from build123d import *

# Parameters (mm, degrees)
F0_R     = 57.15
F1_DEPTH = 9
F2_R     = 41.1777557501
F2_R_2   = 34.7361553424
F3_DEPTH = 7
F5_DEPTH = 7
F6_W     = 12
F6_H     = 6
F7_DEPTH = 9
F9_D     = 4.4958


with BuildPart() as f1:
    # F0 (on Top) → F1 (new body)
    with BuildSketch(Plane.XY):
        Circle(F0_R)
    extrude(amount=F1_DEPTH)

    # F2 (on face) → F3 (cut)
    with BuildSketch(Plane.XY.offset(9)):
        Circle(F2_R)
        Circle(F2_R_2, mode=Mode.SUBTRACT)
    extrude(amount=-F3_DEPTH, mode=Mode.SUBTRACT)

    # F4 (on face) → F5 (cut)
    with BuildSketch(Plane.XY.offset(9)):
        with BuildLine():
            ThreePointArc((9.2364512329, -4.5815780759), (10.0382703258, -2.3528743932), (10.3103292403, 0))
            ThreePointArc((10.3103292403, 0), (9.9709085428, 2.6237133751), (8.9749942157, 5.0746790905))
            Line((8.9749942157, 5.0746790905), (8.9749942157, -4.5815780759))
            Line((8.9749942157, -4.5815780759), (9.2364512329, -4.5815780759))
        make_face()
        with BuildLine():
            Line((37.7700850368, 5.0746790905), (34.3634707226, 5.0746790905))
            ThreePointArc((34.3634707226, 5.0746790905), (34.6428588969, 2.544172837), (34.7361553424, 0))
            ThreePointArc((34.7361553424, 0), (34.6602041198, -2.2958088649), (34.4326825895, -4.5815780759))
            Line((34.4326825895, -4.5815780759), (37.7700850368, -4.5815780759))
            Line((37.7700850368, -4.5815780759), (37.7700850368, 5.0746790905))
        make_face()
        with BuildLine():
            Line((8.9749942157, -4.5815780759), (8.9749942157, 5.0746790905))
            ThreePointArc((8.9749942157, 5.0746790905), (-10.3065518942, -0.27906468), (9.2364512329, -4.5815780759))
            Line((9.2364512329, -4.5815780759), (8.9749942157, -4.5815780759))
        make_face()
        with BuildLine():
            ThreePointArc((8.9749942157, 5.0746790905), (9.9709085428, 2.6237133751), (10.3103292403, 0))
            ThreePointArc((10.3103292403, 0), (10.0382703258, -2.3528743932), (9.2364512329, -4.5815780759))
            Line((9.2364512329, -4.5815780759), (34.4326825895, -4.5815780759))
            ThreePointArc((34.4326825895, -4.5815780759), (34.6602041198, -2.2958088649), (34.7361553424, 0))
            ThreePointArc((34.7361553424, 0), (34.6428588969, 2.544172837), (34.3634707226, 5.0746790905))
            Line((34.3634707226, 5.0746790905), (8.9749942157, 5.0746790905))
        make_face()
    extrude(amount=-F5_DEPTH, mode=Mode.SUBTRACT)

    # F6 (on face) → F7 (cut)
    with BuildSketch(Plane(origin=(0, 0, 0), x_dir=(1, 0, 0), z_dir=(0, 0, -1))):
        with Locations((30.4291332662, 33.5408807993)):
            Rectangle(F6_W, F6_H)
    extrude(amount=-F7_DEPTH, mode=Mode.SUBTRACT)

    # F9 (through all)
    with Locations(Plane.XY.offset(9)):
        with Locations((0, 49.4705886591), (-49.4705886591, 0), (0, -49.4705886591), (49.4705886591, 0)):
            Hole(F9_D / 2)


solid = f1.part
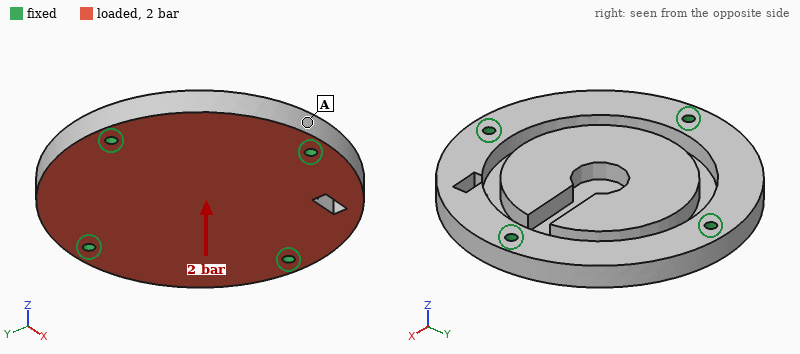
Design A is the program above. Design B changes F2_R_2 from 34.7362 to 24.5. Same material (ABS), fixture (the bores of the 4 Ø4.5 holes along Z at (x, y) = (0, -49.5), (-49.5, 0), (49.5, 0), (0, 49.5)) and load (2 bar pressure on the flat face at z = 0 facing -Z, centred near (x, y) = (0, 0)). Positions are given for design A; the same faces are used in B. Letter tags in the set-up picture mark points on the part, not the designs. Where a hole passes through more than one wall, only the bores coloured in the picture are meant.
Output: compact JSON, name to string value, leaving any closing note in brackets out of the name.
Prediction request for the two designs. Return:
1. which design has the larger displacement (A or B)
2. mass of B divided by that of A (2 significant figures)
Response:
{"which design has the larger displacement": "B", "mass of B divided by that of A": "0.83"}
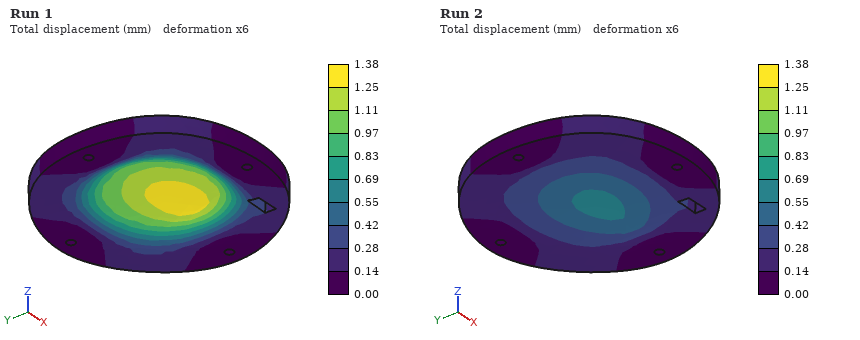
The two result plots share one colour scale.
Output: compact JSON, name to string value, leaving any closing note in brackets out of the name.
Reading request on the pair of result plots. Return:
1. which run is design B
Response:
{"which run is design B": "Run 1"}
